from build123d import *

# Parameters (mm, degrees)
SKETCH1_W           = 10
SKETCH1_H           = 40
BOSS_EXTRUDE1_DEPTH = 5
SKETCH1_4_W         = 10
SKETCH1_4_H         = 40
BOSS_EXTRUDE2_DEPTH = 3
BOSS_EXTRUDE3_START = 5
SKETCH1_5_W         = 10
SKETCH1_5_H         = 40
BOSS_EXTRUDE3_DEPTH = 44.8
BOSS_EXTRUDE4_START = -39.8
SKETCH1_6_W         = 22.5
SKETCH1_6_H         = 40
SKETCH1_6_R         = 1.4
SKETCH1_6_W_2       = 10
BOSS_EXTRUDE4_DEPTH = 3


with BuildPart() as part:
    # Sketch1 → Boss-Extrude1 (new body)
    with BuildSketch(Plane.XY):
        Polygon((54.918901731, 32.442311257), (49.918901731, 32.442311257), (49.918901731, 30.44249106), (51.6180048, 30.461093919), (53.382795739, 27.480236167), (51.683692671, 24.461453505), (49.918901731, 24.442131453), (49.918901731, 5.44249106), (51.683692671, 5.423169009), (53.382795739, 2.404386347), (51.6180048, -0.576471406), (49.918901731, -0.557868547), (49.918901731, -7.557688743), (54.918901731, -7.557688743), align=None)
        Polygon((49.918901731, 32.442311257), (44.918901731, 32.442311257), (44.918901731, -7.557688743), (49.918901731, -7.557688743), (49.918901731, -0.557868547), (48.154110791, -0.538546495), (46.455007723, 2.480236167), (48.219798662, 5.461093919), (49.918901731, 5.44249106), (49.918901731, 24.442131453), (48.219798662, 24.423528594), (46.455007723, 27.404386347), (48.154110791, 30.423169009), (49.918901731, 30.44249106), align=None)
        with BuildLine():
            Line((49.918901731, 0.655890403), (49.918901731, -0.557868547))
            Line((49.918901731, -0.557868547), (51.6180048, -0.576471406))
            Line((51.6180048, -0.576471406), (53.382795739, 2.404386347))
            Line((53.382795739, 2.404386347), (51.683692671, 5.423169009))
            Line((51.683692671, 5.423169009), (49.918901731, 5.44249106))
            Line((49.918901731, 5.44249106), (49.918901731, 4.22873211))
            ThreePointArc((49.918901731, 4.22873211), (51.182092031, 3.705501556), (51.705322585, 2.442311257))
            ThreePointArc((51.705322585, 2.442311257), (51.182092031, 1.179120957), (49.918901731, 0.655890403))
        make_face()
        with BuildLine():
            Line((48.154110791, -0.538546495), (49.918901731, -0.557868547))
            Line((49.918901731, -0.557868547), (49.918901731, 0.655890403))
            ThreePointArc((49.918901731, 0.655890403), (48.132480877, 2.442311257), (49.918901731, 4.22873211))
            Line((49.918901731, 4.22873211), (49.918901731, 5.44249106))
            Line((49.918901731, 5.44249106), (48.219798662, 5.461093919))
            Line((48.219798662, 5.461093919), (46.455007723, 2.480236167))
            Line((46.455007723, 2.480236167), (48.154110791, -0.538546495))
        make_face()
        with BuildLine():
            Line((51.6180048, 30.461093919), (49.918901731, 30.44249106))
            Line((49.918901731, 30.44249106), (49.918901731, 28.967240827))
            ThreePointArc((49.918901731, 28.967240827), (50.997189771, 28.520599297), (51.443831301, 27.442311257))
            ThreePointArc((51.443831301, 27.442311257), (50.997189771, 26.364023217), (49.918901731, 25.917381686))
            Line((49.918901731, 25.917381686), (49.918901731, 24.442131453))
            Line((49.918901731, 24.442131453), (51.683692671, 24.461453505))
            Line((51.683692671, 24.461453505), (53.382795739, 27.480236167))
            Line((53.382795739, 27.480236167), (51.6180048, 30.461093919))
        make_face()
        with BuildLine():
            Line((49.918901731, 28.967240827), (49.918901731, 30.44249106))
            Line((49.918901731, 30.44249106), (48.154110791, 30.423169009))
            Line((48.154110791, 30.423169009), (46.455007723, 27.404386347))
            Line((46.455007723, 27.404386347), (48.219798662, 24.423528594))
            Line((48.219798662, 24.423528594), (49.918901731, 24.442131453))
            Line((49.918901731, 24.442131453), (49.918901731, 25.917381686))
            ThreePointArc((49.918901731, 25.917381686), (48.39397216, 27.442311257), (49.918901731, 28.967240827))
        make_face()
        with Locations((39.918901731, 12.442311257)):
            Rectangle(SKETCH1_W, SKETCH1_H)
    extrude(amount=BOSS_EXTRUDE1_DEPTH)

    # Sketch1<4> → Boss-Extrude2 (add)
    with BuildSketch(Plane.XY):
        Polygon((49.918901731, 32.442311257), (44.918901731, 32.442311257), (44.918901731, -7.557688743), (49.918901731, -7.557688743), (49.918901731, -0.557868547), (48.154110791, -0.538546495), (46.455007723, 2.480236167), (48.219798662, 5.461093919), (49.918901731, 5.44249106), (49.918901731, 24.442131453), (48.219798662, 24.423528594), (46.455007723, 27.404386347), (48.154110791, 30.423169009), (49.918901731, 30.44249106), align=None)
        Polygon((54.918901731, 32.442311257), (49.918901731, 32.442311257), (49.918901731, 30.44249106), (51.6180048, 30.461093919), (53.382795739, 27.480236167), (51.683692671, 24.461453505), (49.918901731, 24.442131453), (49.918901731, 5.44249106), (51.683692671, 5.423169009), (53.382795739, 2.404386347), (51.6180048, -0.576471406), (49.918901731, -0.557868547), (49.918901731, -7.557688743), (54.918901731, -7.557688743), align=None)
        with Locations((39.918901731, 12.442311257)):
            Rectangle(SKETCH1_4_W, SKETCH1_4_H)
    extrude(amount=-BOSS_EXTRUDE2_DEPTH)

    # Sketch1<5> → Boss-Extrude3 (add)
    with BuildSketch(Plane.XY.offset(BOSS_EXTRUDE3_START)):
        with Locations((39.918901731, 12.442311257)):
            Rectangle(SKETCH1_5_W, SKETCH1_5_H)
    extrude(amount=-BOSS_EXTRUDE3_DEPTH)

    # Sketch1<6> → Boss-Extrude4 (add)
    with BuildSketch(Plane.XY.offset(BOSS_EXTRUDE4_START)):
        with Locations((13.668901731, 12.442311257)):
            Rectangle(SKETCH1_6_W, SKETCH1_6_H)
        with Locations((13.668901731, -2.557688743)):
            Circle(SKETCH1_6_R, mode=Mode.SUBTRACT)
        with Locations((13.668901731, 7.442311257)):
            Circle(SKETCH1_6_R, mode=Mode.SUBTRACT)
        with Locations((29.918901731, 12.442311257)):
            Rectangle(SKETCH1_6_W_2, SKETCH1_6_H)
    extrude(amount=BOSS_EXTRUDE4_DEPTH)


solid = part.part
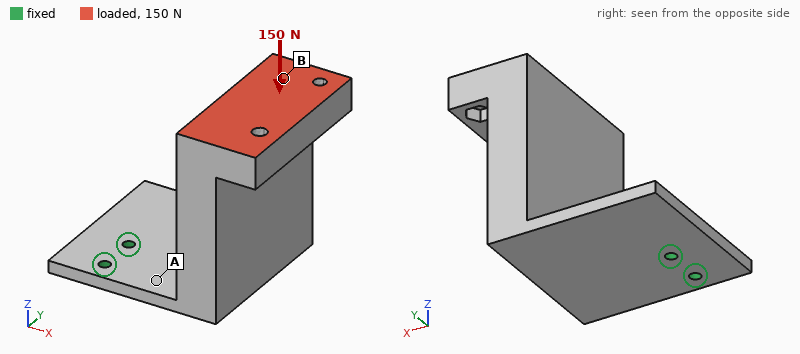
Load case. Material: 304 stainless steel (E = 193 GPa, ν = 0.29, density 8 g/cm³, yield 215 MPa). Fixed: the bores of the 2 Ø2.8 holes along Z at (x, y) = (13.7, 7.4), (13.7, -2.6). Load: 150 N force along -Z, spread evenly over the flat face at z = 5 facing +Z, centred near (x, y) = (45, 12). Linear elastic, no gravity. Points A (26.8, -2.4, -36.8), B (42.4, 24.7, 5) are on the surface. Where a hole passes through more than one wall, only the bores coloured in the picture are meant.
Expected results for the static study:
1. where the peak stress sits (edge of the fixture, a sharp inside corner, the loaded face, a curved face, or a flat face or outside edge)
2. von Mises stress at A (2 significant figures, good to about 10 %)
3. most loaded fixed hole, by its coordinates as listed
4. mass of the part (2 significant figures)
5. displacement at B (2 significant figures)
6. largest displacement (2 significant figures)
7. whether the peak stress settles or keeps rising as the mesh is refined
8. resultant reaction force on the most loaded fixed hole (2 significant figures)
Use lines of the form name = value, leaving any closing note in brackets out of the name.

where the peak stress sits = edge of the fixture
von Mises stress at A = 55 MPa
most loaded fixed hole, by its coordinates as listed = (13.7, 7.4)
mass of the part = 200 g
displacement at B = 0.23 mm
largest displacement = 0.27 mm
whether the peak stress settles or keeps rising as the mesh is refined = keeps rising
resultant reaction force on the most loaded fixed hole = 160 N
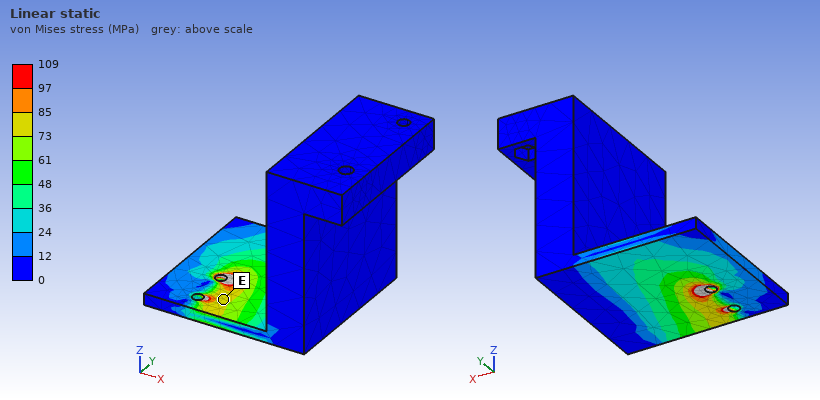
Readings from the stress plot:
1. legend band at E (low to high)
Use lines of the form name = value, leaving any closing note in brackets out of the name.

legend band at E = 73 to 85 MPa
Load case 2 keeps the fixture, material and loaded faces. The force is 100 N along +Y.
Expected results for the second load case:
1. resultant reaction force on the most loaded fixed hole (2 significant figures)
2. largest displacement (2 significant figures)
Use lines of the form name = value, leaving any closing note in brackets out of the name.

resultant reaction force on the most loaded fixed hole = 380 N
largest displacement = 0.14 mm
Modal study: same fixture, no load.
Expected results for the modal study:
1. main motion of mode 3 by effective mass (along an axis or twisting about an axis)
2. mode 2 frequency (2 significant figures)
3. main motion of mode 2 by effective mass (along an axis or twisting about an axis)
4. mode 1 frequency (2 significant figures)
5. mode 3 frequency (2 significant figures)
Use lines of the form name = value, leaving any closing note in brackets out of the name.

main motion of mode 3 by effective mass = along Z
mode 2 frequency = 530 Hz
main motion of mode 2 by effective mass = along Y
mode 1 frequency = 310 Hz
mode 3 frequency = 1600 Hz
